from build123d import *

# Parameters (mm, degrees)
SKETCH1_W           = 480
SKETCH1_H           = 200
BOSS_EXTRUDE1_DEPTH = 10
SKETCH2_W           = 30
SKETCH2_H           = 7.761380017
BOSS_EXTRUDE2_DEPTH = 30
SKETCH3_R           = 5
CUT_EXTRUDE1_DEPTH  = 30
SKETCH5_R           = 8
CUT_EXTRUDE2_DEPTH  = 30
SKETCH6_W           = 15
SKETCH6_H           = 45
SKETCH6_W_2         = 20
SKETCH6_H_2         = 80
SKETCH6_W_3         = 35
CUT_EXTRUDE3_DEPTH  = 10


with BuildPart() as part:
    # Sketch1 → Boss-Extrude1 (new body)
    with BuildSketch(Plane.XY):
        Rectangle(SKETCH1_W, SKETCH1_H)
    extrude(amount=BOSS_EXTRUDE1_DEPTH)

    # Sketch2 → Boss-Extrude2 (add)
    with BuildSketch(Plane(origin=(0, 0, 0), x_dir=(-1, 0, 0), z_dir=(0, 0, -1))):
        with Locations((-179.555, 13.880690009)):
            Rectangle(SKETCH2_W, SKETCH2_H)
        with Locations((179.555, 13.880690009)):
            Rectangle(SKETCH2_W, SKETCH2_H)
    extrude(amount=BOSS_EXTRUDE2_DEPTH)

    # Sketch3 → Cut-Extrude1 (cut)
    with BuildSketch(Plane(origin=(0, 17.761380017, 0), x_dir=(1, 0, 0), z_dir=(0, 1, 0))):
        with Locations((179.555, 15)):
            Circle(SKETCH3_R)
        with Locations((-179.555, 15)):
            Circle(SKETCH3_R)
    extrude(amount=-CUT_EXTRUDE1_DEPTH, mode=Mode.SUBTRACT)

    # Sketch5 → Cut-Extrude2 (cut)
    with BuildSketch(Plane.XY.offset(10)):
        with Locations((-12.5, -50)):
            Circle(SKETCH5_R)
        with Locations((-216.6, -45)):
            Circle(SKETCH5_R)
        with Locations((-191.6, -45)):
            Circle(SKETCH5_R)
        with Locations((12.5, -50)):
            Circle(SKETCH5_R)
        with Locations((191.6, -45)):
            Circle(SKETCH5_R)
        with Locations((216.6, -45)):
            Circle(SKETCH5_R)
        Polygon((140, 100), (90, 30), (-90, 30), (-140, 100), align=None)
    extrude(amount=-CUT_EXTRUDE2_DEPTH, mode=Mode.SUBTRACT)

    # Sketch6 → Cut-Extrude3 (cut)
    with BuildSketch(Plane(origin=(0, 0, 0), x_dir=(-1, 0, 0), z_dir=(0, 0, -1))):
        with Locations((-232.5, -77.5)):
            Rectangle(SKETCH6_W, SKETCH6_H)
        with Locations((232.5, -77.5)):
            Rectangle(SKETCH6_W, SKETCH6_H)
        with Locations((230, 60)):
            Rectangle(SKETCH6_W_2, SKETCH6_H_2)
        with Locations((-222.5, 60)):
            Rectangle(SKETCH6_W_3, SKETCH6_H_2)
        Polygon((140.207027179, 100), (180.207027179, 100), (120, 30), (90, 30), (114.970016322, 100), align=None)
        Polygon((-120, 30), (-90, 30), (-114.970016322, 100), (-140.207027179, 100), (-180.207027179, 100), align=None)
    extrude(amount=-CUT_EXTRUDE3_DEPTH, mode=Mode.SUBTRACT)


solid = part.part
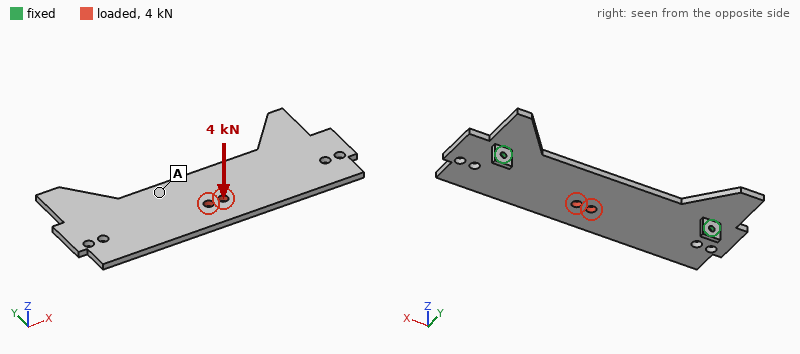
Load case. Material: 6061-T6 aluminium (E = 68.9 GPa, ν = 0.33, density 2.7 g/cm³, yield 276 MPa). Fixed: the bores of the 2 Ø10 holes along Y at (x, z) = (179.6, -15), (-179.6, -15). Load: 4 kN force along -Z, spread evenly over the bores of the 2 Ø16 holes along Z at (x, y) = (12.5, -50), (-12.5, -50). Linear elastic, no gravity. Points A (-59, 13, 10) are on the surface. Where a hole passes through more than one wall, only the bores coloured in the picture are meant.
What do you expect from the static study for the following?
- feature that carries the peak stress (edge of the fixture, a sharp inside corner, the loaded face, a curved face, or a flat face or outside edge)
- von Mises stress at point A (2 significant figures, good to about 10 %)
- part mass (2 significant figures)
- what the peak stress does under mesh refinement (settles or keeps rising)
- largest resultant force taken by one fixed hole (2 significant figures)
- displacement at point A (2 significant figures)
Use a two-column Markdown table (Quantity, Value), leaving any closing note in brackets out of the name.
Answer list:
| Quantity | Value |
|---|---|
| feature that carries the peak stress | edge of the fixture |
| von Mises stress at point A | 45 MPa |
| part mass | 1.9 kg |
| what the peak stress does under mesh refinement | keeps rising |
| largest resultant force taken by one fixed hole | 5.1 kN |
| displacement at point A | 1.2 mm |
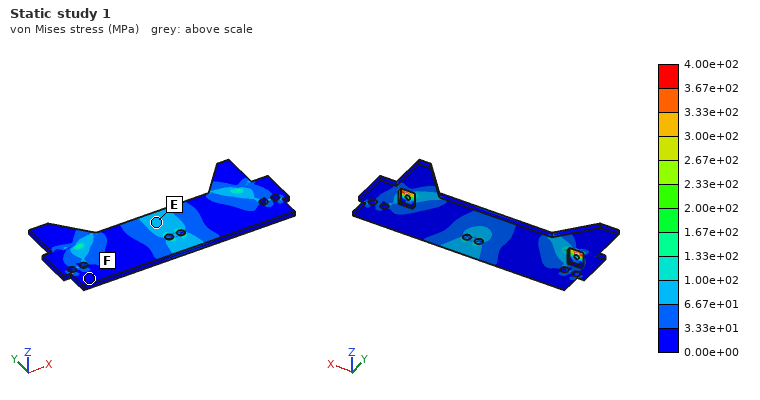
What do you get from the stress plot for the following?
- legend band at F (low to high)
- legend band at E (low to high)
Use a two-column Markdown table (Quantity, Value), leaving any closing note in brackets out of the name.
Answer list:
| Quantity | Value |
|---|---|
| legend band at F | 0.00e+00 to 3.33e+01 MPa |
| legend band at E | 6.67e+01 to 1.00e+02 MPa |
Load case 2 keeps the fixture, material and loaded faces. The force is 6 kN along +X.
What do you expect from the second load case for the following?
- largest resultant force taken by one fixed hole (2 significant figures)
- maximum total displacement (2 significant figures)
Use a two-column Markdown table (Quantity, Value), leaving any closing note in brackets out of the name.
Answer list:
| Quantity | Value |
|---|---|
| largest resultant force taken by one fixed hole | 3.2 kN |
| maximum total displacement | 0.11 mm |
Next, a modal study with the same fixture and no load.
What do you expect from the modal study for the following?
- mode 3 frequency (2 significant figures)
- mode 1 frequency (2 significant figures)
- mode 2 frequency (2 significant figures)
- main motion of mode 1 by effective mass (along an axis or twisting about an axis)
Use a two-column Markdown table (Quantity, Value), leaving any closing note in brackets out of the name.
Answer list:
| Quantity | Value |
|---|---|
| mode 3 frequency | 430 Hz |
| mode 1 frequency | 180 Hz |
| mode 2 frequency | 380 Hz |
| main motion of mode 1 by effective mass | along Z |
